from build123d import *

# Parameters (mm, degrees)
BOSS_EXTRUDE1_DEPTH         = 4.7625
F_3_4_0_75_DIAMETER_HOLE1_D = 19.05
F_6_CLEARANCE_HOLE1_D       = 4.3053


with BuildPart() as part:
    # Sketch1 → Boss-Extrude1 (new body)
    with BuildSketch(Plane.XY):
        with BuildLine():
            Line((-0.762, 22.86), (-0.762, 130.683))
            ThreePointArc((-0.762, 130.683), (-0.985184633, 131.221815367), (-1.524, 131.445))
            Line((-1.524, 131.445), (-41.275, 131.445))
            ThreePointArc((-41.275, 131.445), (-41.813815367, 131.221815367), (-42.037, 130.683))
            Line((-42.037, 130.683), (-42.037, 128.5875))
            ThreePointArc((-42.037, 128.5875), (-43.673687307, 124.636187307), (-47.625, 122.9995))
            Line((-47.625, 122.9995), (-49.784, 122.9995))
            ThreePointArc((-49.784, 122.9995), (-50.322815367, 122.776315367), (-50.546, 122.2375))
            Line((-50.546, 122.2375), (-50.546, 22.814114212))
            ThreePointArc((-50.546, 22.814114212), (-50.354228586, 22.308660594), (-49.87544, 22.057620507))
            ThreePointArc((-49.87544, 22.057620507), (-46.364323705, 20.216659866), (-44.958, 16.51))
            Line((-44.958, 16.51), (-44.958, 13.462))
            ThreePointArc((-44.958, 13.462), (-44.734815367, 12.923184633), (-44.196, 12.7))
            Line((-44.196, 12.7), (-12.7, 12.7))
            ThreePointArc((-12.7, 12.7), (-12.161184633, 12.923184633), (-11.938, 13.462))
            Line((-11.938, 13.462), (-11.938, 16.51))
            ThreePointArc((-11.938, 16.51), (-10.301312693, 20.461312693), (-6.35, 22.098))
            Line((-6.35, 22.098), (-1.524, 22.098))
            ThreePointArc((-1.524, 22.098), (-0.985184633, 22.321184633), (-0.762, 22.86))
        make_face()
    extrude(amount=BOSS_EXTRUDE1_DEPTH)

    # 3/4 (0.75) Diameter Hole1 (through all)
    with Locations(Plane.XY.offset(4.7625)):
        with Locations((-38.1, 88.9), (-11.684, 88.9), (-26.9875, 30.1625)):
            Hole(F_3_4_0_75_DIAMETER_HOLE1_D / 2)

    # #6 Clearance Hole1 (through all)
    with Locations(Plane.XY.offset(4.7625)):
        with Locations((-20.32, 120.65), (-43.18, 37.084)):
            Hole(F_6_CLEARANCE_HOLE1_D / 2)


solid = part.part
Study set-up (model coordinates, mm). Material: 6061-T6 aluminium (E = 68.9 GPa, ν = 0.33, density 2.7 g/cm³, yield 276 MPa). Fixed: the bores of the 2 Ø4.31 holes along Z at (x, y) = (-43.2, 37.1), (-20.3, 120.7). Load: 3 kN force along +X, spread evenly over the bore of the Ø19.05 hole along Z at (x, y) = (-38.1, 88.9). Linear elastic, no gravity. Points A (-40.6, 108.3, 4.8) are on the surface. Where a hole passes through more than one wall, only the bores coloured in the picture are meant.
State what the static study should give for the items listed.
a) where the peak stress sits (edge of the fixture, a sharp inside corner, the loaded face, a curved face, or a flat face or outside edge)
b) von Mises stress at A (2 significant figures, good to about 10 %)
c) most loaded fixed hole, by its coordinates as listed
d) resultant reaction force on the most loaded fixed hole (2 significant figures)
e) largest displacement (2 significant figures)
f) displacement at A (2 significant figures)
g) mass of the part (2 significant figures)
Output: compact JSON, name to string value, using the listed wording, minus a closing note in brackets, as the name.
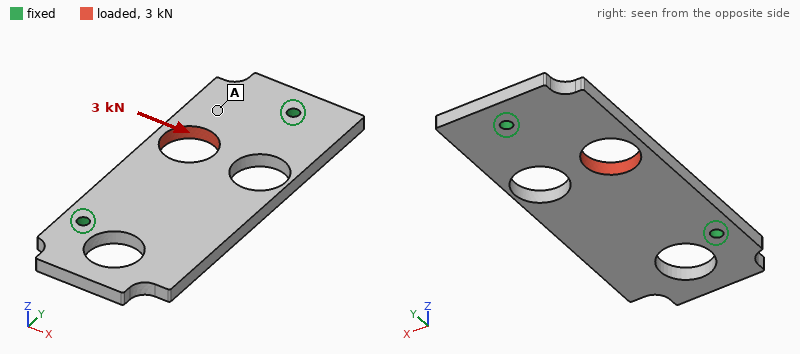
{"where the peak stress sits": "a curved face", "von Mises stress at A": "19 MPa", "most loaded fixed hole, by its coordinates as listed": "(-20.3, 120.7)", "resultant reaction force on the most loaded fixed hole": "1.8 kN", "largest displacement": "41 µm", "displacement at A": "21 µm", "mass of the part": "62 g"}
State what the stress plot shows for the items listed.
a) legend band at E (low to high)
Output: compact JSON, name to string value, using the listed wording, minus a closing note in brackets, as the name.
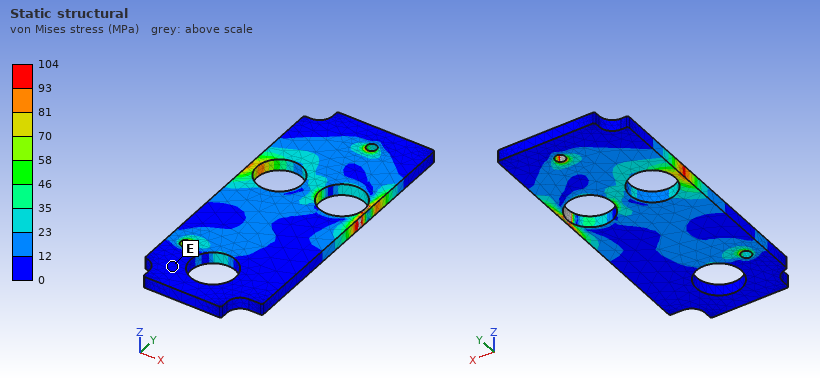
{"legend band at E": "0 to 12 MPa"}
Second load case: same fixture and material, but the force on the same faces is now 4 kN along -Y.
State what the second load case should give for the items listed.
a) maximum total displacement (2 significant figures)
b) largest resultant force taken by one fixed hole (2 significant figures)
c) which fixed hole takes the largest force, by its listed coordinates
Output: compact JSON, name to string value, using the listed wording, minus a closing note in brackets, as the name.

{"maximum total displacement": "29 µm", "largest resultant force taken by one fixed hole": "2.3 kN", "which fixed hole takes the largest force, by its listed coordinates": "(-20.3, 120.7)"}
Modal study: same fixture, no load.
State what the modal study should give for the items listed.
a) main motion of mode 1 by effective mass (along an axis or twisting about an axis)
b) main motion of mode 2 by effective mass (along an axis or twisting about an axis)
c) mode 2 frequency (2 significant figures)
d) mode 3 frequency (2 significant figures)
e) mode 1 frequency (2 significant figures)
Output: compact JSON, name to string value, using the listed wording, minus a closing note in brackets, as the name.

{"main motion of mode 1 by effective mass": "along Z", "main motion of mode 2 by effective mass": "along Z", "mode 2 frequency": "2700 Hz", "mode 3 frequency": "3600 Hz", "mode 1 frequency": "1700 Hz"}
